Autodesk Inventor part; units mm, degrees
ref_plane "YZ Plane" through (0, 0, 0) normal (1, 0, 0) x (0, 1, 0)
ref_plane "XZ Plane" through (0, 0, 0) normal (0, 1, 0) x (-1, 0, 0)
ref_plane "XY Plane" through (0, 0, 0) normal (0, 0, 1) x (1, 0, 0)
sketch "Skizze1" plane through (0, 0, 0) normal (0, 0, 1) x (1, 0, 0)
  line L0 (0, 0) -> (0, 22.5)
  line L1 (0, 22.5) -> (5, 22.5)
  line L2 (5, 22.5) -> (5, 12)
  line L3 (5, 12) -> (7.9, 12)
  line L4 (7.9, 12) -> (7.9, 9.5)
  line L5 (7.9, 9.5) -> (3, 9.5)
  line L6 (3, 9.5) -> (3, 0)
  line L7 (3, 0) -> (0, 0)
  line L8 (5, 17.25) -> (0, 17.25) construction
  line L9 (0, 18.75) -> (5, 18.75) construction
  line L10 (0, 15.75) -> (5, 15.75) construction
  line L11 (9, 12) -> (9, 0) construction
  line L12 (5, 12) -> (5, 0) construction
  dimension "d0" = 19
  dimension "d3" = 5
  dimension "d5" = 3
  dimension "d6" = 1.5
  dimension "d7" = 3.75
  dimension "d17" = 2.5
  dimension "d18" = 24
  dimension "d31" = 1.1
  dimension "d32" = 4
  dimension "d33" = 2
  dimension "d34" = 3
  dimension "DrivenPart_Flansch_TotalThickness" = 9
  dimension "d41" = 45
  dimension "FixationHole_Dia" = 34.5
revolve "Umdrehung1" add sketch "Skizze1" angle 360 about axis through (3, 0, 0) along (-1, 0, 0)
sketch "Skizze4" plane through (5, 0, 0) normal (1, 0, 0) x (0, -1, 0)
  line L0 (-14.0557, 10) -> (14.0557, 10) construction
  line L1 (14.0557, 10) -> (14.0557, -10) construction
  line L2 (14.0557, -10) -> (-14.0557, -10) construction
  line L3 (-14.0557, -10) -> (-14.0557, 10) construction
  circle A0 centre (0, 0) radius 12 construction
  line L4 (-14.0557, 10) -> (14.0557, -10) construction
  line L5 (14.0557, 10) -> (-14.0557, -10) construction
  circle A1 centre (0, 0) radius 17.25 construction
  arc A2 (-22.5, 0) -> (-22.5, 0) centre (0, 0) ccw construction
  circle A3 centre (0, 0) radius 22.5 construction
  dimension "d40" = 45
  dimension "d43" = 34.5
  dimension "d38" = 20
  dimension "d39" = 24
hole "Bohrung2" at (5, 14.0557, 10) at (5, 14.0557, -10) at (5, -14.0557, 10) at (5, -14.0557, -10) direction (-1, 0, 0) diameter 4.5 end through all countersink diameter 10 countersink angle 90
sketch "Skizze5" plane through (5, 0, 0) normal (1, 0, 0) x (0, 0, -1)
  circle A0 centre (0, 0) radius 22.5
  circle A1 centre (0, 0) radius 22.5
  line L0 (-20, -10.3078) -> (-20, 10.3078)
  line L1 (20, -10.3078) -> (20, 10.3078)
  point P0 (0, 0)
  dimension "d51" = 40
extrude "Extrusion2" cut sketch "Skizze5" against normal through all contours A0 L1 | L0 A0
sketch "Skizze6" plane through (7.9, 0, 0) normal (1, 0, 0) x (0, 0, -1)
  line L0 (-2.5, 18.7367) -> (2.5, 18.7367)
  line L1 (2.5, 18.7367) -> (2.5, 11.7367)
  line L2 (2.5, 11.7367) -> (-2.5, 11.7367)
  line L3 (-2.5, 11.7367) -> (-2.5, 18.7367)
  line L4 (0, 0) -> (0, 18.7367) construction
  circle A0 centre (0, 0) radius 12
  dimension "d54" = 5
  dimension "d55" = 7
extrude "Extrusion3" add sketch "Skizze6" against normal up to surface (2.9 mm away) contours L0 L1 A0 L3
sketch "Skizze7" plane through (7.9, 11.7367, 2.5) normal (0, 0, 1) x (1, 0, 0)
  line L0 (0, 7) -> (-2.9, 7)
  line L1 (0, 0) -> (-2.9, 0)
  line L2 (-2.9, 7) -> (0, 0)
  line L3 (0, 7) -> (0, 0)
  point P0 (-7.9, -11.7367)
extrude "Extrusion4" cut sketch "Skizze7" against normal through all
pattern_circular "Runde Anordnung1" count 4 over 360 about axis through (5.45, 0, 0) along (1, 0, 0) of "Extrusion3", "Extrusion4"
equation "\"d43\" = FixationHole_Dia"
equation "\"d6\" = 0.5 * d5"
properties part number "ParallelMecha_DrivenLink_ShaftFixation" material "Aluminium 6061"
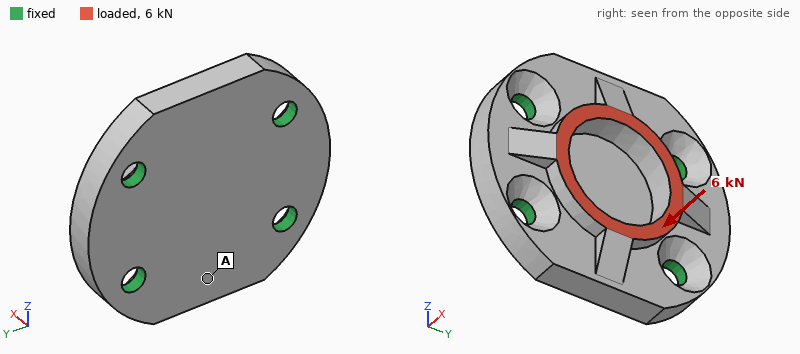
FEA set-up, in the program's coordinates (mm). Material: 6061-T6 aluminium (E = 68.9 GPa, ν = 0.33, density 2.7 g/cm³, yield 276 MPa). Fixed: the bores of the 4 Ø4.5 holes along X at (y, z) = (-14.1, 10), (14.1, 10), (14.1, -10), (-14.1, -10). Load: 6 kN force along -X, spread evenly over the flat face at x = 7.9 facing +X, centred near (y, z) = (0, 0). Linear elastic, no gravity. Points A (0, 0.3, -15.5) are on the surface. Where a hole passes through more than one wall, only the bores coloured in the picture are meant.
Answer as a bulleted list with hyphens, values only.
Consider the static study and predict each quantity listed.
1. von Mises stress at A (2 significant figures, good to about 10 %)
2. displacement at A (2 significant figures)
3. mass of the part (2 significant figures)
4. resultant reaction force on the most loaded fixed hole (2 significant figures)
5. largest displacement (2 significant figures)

- 40 MPa
- 22 µm
- 19 g
- 1.7 kN
- 27 µm
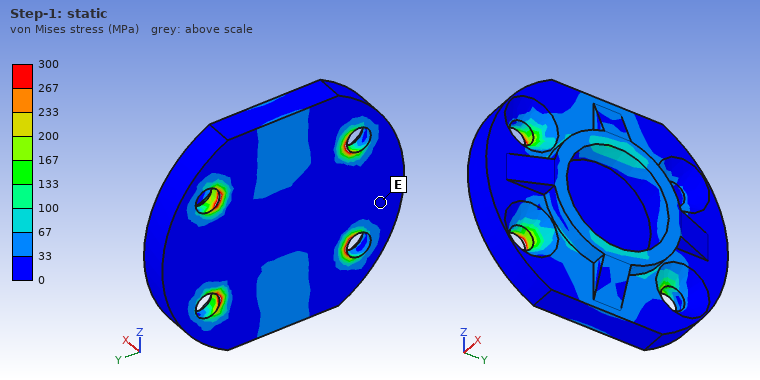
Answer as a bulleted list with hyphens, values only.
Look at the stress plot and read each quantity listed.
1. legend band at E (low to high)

- 0 to 33 MPa
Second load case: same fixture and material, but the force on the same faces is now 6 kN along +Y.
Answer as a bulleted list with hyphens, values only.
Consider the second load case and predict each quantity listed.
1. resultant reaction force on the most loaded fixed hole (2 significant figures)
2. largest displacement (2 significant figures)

- 1.7 kN
- 24 µm
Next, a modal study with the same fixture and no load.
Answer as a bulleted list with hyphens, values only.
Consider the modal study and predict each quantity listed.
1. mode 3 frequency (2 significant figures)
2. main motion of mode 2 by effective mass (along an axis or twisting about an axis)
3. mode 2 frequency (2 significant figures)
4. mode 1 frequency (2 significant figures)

- 29 kHz
- twisting about Y
- 20 kHz
- 19 kHz
